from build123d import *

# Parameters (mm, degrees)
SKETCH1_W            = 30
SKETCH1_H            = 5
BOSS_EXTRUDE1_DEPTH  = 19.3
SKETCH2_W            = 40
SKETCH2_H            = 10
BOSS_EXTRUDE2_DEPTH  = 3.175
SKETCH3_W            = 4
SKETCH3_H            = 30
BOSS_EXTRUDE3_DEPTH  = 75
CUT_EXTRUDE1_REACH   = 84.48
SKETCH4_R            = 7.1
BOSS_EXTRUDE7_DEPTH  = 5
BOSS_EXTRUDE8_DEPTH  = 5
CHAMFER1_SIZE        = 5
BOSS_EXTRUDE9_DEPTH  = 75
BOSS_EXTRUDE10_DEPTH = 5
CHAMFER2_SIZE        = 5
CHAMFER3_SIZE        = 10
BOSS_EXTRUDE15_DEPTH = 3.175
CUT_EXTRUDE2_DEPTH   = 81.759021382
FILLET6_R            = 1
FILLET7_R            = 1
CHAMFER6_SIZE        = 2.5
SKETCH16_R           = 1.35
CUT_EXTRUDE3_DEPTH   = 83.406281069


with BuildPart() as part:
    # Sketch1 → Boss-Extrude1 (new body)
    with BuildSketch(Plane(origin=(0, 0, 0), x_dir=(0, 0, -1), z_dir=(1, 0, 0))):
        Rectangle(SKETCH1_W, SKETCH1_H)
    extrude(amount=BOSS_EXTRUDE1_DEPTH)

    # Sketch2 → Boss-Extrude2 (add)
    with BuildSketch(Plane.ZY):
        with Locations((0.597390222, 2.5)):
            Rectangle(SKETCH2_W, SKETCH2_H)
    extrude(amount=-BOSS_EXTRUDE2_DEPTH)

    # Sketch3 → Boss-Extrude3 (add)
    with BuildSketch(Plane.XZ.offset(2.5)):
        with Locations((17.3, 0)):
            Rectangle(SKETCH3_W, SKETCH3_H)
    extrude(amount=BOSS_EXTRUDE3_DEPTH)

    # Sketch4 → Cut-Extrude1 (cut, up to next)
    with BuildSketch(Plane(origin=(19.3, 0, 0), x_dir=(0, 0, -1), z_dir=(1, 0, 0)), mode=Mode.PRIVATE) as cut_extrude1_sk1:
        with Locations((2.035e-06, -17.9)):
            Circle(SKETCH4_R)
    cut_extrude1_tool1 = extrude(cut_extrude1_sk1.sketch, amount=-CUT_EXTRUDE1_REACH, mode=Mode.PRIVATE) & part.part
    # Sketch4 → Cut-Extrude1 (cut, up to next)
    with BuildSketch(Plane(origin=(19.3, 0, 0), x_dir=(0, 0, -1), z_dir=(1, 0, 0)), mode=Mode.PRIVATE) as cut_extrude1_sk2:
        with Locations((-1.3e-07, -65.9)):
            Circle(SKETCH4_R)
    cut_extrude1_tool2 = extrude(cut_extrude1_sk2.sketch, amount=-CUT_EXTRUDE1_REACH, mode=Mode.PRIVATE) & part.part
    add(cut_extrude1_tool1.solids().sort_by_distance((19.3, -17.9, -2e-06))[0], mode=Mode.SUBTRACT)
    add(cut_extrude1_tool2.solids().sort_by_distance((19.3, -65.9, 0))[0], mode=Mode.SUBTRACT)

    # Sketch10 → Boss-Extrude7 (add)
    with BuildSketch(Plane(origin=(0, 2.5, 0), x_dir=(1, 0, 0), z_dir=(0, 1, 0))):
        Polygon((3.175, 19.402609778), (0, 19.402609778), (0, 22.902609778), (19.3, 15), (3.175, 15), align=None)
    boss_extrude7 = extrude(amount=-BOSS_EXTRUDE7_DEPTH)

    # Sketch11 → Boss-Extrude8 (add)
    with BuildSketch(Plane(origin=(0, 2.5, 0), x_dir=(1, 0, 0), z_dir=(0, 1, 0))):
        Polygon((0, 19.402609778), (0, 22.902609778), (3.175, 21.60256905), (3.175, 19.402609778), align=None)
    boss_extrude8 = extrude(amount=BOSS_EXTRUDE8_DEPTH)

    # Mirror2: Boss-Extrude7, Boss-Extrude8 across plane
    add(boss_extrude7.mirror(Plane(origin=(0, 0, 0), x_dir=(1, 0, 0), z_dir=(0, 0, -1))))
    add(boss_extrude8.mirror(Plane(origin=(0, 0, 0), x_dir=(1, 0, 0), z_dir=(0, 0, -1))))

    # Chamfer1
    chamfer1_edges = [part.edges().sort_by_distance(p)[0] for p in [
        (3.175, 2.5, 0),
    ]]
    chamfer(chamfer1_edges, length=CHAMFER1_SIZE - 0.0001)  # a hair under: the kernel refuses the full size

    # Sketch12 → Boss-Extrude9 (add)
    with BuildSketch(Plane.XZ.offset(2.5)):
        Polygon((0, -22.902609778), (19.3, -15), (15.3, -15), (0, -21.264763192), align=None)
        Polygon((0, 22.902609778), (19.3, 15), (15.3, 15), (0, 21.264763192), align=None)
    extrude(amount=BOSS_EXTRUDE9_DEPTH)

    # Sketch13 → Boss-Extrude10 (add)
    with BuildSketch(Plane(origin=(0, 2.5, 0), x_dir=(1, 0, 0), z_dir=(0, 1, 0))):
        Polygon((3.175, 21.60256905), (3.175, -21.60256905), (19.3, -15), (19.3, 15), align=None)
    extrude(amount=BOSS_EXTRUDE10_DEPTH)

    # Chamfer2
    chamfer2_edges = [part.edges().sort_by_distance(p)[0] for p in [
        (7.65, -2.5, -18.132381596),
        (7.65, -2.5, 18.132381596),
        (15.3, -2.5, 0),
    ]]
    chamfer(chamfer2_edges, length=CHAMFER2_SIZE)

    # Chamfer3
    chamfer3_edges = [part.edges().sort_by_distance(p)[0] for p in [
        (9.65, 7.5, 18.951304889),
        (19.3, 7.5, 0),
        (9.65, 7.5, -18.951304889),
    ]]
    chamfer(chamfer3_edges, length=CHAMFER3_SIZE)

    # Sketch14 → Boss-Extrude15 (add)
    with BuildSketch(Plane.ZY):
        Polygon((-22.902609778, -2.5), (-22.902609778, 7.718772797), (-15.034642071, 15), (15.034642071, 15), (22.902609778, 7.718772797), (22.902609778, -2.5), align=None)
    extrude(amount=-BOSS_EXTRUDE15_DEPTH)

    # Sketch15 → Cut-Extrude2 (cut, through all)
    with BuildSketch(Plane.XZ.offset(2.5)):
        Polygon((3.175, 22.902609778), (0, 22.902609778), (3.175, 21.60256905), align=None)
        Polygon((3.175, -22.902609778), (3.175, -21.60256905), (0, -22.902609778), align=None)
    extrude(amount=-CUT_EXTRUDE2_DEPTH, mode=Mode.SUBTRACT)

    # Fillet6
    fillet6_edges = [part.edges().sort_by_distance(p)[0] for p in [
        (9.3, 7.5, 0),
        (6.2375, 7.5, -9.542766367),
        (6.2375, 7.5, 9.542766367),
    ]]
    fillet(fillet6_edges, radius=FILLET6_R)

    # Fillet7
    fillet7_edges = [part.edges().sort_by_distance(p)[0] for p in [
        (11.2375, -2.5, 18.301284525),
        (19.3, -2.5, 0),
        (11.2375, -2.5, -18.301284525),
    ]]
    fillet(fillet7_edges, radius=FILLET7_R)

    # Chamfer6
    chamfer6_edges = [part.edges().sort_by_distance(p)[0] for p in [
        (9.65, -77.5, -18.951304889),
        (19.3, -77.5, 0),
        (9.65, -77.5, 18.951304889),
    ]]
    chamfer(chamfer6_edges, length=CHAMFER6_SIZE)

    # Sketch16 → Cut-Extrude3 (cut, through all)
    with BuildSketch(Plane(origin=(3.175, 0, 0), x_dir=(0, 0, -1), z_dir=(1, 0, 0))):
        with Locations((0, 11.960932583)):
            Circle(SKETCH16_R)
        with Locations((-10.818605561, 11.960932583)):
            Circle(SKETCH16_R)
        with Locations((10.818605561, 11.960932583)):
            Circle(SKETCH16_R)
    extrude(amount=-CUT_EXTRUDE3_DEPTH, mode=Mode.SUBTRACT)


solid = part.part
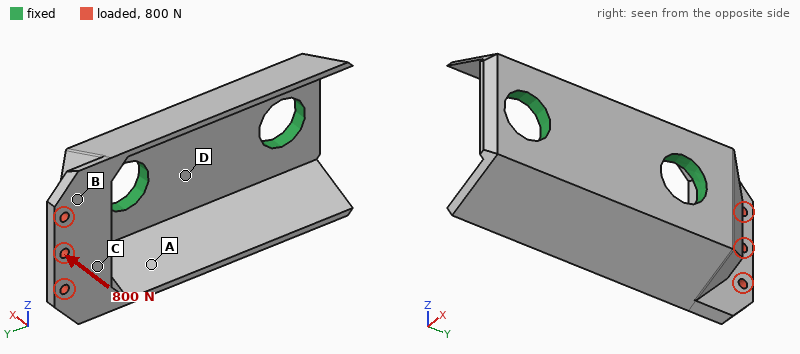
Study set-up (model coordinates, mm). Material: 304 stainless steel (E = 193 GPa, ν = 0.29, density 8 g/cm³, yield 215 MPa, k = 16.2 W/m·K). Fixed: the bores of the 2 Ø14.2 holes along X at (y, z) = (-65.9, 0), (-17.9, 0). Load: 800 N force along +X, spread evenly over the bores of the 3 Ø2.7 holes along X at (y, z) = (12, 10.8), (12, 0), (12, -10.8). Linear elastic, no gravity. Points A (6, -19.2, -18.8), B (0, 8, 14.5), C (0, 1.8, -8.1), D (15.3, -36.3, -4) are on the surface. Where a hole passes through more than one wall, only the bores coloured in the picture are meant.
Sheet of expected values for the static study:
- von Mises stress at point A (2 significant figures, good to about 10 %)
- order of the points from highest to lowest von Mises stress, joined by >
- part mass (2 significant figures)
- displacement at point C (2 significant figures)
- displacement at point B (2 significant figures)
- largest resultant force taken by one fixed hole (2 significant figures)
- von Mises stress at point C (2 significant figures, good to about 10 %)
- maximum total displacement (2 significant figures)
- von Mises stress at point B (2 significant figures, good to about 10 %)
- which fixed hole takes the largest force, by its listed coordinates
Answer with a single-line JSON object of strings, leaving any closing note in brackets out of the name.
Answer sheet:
{"von Mises stress at point A": "23 MPa", "order of the points from highest to lowest von Mises stress, joined by >": "B > A > C > D", "part mass": "140 g", "displacement at point C": "17 µm", "displacement at point B": "21 µm", "largest resultant force taken by one fixed hole": "1.1 kN", "von Mises stress at point C": "13 MPa", "maximum total displacement": "33 µm", "von Mises stress at point B": "35 MPa", "which fixed hole takes the largest force, by its listed coordinates": "(-17.9, 0)"}
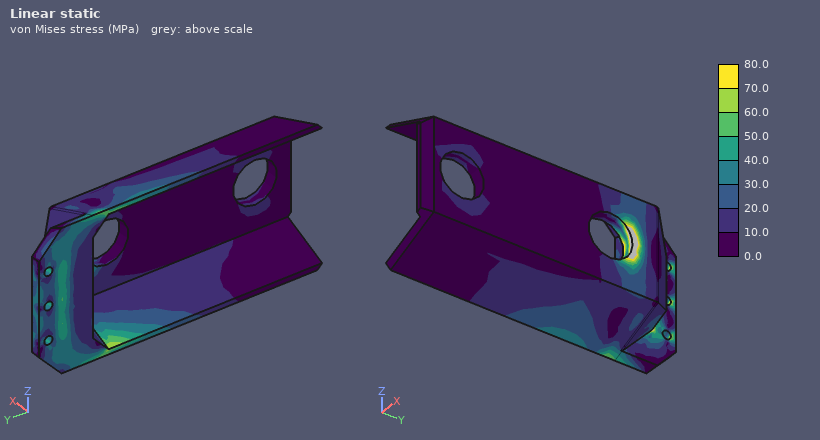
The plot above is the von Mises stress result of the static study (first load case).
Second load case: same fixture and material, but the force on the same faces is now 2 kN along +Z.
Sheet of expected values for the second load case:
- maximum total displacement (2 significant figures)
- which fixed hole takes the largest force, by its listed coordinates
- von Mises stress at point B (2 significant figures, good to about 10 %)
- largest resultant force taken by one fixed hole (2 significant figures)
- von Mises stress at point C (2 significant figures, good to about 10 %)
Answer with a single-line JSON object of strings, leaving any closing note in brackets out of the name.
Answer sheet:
{"maximum total displacement": "48 µm", "which fixed hole takes the largest force, by its listed coordinates": "(-17.9, 0)", "von Mises stress at point B": "24 MPa", "largest resultant force taken by one fixed hole": "2.3 kN", "von Mises stress at point C": "21 MPa"}
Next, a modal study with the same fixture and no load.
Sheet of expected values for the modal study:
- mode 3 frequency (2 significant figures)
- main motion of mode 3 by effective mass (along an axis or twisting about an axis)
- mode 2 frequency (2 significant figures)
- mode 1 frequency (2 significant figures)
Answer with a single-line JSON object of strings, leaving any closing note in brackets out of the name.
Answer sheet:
{"mode 3 frequency": "4900 Hz", "main motion of mode 3 by effective mass": "along Z", "mode 2 frequency": "4100 Hz", "mode 1 frequency": "4100 Hz"}
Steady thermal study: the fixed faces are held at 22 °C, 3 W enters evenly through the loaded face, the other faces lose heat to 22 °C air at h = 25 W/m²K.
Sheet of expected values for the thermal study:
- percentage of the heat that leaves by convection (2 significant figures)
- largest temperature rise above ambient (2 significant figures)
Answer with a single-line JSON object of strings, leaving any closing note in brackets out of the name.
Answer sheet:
{"percentage of the heat that leaves by convection": "43 %", "largest temperature rise above ambient": "29 K"}
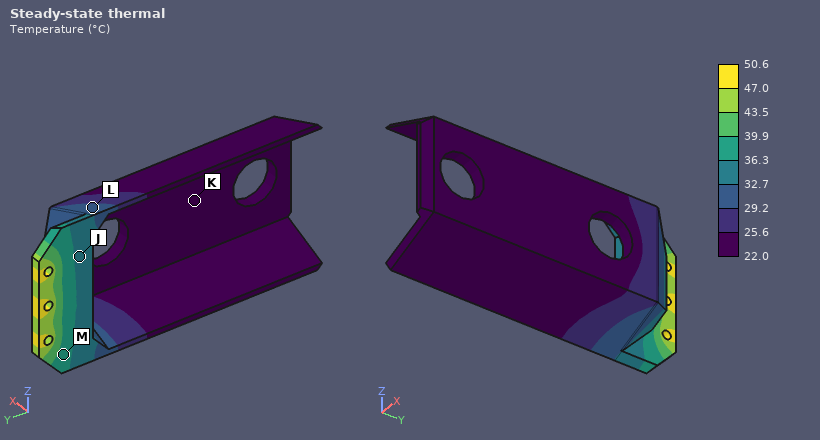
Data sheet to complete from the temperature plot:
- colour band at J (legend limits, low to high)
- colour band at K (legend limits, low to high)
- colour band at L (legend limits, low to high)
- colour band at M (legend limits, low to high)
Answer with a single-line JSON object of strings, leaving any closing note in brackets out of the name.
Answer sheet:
{"colour band at J": "32.7 to 36.3 °C", "colour band at K": "22.0 to 25.6 °C", "colour band at L": "29.2 to 32.7 °C", "colour band at M": "36.3 to 39.9 °C"}
